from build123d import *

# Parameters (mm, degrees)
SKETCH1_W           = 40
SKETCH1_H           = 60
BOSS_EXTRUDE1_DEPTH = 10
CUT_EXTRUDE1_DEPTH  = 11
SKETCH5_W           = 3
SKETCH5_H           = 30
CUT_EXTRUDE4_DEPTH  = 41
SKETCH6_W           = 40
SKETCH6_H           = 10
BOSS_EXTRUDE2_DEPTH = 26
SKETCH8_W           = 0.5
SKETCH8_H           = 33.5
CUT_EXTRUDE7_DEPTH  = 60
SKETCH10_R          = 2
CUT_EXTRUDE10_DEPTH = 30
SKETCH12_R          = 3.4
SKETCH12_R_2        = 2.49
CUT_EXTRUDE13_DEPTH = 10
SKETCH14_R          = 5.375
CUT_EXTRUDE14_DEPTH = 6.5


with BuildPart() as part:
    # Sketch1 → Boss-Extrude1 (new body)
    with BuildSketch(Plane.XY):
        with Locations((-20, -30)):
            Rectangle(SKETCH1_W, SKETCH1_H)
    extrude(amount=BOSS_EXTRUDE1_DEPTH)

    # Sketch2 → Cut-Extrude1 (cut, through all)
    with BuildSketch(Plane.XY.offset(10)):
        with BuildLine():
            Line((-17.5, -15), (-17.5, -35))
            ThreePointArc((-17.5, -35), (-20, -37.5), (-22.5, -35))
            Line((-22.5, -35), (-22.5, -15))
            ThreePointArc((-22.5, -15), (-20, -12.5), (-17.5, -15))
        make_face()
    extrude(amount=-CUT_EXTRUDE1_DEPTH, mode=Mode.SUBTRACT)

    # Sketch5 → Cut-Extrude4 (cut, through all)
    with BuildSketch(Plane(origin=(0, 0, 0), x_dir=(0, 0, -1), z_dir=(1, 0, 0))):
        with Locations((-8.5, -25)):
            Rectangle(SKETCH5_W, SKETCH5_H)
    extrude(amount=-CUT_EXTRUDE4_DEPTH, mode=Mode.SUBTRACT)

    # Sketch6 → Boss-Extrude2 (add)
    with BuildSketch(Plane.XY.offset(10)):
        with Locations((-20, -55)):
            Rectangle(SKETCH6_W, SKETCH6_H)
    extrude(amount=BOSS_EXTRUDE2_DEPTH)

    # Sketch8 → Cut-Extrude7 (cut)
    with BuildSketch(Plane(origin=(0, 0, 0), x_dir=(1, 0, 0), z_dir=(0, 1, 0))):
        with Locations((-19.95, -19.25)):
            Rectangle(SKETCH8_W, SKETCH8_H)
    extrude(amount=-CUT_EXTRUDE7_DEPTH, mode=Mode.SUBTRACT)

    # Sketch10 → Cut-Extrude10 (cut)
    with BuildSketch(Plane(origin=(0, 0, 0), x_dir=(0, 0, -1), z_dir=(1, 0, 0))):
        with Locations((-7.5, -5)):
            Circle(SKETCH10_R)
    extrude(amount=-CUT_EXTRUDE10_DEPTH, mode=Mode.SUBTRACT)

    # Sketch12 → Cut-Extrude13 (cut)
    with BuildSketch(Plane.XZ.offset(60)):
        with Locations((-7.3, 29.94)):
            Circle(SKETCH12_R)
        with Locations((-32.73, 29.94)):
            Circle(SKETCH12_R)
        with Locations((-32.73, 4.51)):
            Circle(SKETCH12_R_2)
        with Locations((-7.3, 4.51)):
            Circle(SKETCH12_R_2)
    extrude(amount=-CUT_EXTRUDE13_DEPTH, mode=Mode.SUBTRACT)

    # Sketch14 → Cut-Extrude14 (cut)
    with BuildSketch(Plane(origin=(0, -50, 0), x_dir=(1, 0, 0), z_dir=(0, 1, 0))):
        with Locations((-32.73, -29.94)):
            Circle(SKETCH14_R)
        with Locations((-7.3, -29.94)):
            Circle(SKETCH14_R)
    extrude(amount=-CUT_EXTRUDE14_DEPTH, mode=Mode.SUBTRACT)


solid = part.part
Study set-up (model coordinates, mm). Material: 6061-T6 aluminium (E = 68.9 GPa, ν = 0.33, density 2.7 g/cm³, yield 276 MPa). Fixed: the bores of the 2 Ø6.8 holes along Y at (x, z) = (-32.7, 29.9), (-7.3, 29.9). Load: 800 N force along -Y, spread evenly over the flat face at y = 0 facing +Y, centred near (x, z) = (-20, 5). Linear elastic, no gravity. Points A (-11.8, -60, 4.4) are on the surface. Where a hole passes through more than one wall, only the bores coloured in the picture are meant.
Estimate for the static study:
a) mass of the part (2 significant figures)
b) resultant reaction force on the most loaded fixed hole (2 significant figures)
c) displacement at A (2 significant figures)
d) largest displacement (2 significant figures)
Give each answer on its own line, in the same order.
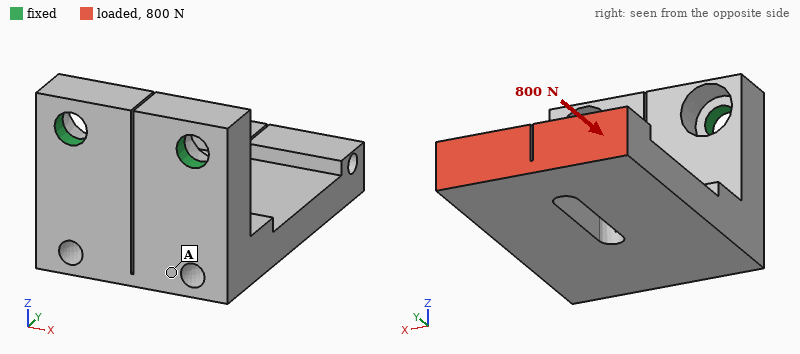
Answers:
74 g
400 N
0.065 mm
0.17 mm
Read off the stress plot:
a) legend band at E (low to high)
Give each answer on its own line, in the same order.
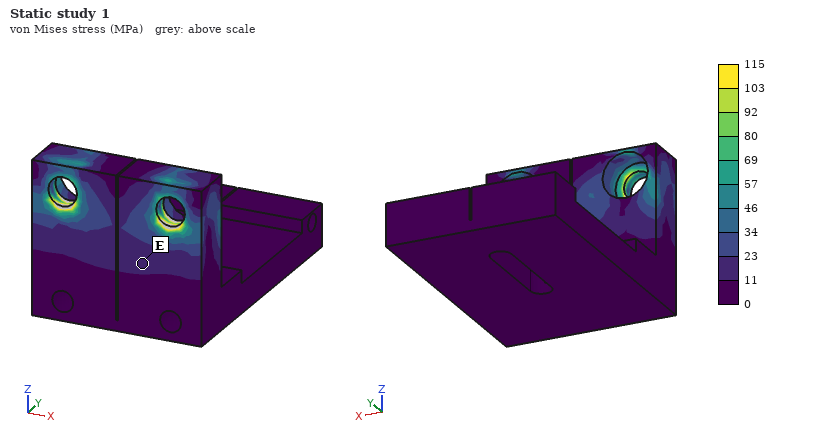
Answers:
11 to 23 MPa
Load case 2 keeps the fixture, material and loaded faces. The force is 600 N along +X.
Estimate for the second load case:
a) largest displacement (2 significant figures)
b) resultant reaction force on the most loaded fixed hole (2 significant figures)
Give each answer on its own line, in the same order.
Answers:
0.22 mm
1.0 kN
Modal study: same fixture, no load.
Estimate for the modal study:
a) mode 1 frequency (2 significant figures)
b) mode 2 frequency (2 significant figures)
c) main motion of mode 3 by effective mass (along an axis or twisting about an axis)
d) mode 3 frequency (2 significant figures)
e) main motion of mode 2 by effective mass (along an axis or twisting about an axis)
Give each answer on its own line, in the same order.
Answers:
1200 Hz
2100 Hz
along Y
3800 Hz
along X
